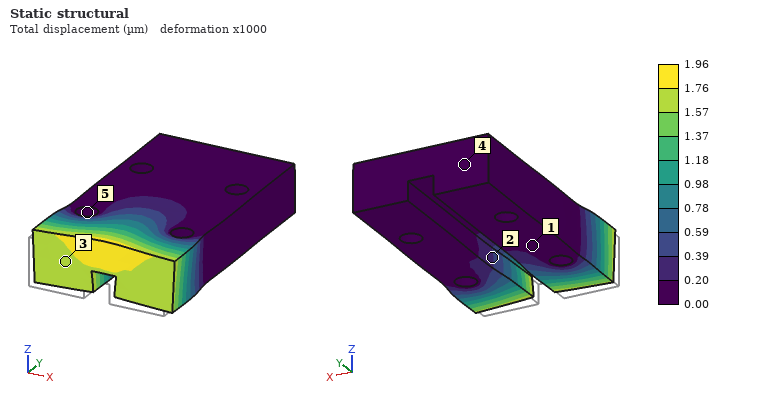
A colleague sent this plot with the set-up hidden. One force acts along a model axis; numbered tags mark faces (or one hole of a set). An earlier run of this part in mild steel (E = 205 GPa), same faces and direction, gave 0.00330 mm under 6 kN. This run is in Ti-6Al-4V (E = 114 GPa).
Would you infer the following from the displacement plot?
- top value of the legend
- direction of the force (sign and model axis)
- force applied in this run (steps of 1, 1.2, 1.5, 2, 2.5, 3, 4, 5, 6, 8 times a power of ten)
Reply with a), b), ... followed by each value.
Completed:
a) 1.96 µm
b) +Y
c) 2 kN
